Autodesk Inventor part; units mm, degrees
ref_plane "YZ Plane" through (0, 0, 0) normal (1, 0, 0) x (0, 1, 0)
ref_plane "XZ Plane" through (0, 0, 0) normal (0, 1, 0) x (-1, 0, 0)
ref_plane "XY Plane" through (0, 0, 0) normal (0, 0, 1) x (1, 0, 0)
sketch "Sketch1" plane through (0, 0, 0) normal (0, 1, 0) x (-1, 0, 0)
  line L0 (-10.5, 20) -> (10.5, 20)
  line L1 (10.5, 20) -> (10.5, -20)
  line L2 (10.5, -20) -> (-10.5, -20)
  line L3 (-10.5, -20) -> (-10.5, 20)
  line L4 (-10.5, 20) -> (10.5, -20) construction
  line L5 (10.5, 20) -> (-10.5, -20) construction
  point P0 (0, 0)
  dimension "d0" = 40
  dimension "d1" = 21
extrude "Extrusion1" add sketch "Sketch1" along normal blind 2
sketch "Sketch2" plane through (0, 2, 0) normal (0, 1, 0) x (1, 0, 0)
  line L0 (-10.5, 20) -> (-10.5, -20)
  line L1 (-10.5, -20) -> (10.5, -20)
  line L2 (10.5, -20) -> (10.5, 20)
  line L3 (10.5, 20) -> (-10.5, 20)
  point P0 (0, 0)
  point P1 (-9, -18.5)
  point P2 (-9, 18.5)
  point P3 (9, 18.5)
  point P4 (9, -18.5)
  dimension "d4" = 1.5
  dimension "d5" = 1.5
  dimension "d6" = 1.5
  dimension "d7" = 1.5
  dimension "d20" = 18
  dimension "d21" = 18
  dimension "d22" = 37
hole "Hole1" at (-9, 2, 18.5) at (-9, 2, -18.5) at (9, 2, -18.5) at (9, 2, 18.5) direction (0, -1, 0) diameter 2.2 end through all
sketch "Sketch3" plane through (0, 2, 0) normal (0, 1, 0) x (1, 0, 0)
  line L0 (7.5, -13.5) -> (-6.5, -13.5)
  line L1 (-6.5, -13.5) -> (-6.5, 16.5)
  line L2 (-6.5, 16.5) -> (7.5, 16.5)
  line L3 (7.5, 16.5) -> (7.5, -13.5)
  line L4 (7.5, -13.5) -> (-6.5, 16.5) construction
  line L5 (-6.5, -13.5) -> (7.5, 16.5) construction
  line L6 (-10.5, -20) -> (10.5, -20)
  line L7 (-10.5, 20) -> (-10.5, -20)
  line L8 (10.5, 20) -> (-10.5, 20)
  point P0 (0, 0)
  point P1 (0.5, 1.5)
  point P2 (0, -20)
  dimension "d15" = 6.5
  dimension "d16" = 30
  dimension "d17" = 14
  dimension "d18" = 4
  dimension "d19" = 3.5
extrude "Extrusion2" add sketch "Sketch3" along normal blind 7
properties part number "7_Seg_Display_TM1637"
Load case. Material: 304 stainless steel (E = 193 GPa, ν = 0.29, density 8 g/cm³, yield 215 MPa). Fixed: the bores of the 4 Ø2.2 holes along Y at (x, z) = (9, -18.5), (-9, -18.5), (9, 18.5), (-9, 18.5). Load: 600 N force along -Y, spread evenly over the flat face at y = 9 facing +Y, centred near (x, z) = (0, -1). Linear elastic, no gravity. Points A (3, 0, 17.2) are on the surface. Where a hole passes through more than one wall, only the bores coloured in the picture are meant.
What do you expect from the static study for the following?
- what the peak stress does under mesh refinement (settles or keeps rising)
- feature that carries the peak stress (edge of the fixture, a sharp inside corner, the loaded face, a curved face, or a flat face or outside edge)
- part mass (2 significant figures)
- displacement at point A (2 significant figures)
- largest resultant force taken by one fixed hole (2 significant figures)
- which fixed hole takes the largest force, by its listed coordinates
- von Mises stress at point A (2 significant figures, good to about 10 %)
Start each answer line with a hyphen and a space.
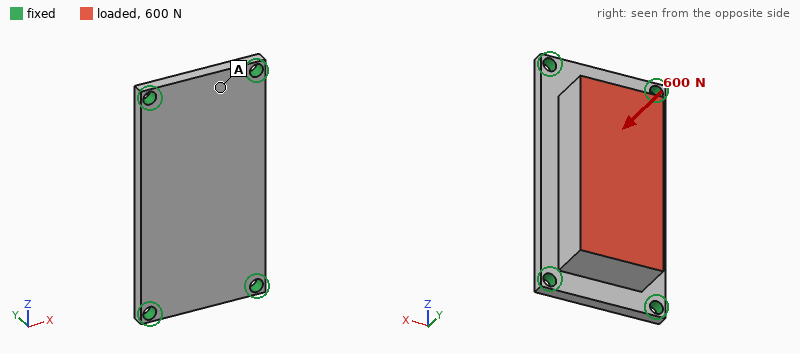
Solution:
- keeps rising
- edge of the fixture
- 37 g
- 2.8 µm
- 210 N
- (9, -18.5)
- 15 MPa
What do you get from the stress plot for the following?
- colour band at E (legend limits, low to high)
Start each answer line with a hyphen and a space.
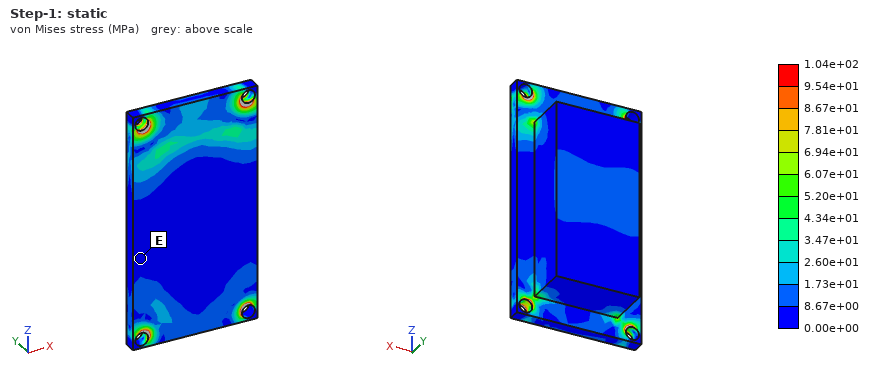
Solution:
- 0.00e+00 to 8.67e+00 MPa
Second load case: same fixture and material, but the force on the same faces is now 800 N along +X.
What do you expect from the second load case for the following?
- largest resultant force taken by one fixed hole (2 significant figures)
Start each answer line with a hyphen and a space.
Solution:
- 420 N
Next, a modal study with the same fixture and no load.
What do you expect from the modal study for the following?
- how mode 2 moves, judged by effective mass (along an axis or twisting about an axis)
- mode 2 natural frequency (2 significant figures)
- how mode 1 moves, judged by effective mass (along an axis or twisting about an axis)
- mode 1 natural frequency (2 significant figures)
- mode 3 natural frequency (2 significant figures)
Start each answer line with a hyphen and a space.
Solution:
- along X
- 14 kHz
- along Y
- 9800 Hz
- 20 kHz
